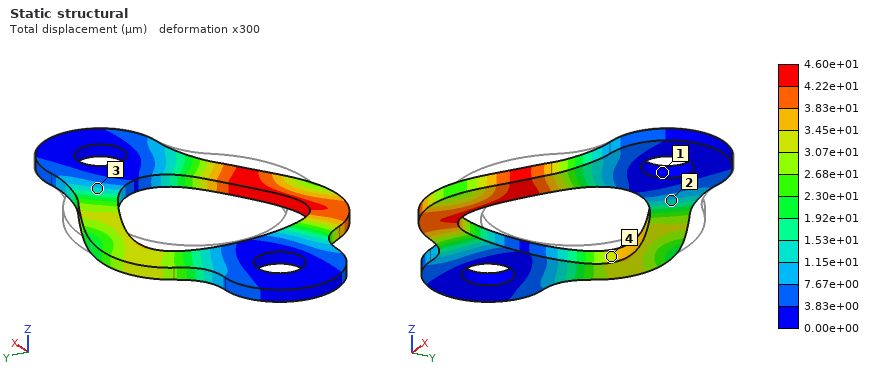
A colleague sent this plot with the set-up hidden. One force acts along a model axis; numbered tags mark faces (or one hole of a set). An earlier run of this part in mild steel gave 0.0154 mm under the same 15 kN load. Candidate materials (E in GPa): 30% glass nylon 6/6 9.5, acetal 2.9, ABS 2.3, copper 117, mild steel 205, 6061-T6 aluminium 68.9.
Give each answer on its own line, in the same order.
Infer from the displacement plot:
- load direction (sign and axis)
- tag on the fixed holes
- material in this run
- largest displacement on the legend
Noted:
-X
1
6061-T6 aluminium
4.60e+01 µm
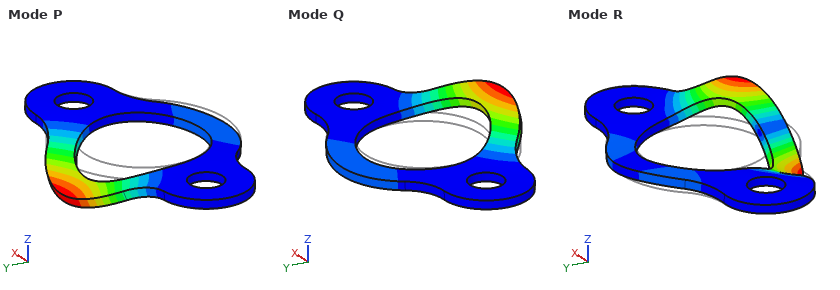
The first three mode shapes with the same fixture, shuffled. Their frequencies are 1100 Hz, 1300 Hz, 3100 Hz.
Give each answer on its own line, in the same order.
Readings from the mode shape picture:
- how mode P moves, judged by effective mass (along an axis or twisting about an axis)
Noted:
along Z
